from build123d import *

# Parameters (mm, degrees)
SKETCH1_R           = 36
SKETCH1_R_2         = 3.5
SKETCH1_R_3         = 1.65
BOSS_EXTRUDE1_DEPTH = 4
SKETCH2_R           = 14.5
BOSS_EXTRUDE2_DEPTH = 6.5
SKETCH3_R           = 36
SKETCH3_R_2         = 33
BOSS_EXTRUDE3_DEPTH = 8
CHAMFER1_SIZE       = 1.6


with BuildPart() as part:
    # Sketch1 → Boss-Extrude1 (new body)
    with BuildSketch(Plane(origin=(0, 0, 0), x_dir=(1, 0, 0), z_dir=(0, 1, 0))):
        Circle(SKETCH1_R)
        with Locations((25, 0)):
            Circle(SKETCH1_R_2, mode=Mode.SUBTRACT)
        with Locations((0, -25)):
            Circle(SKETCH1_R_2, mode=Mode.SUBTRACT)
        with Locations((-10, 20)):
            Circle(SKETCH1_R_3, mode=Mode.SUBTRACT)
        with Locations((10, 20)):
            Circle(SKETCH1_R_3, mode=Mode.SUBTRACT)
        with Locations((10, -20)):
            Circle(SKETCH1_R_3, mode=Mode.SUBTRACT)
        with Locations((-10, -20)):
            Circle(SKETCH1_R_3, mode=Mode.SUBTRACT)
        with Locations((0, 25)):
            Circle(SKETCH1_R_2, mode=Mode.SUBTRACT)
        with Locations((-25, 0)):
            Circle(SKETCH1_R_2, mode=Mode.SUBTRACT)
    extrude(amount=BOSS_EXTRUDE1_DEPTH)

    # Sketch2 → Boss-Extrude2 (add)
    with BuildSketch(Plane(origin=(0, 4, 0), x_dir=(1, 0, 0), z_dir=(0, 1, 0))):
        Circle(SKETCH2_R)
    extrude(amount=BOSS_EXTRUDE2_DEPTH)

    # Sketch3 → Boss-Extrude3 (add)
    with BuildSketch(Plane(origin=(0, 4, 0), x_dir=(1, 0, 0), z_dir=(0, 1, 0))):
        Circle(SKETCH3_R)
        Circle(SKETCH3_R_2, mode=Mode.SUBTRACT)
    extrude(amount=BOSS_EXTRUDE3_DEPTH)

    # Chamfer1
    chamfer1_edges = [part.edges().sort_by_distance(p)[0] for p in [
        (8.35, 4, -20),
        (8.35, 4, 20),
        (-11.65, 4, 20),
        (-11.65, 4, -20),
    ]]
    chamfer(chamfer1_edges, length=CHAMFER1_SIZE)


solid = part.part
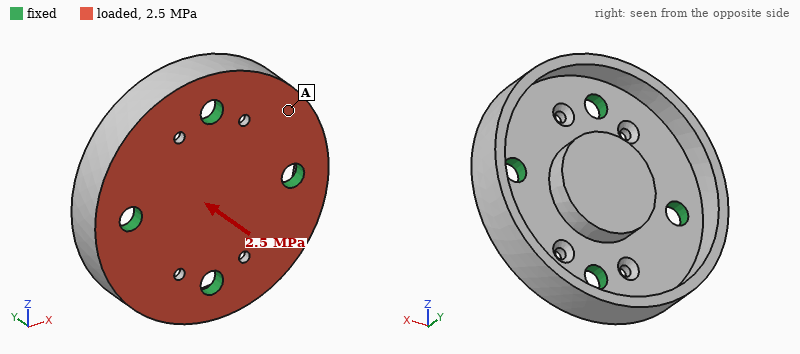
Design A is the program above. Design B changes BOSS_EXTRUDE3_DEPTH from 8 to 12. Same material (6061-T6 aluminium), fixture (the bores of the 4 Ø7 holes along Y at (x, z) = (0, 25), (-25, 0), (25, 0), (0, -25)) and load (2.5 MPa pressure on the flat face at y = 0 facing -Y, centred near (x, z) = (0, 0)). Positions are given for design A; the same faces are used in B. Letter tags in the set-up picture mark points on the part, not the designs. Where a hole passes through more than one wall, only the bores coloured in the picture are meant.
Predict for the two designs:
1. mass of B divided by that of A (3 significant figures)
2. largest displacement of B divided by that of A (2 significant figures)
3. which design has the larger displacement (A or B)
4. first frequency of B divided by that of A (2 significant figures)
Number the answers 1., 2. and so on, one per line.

1. 1.10
2. 0.78
3. A
4. 0.82
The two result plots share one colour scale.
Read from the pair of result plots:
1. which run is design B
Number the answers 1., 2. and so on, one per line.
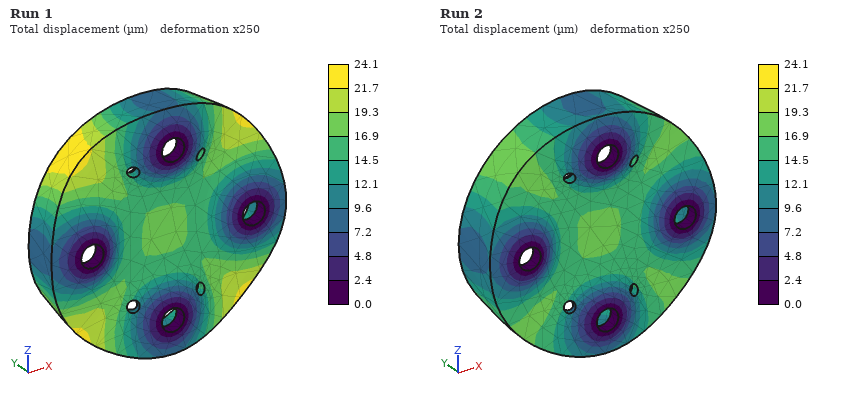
1. Run 2
